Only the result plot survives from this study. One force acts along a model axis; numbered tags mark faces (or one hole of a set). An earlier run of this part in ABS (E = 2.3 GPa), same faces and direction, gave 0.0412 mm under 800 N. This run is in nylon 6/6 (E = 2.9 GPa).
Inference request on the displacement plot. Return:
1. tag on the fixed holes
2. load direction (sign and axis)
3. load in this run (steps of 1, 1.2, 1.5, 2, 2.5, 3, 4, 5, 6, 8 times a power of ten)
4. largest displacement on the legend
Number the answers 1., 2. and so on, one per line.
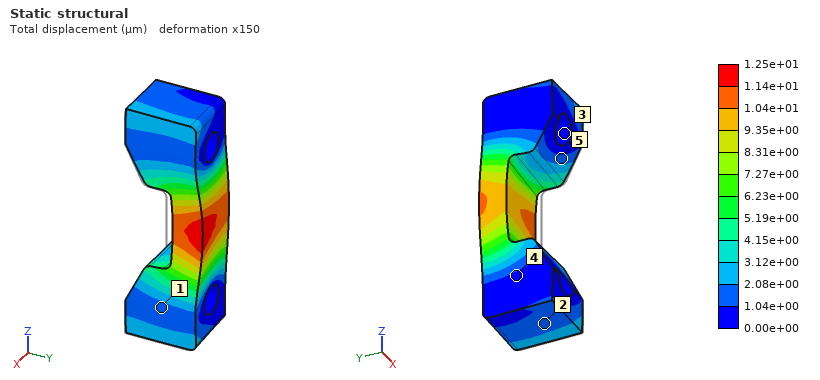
1. 3
2. -X
3. 300 N
4. 1.25e+01 µm
